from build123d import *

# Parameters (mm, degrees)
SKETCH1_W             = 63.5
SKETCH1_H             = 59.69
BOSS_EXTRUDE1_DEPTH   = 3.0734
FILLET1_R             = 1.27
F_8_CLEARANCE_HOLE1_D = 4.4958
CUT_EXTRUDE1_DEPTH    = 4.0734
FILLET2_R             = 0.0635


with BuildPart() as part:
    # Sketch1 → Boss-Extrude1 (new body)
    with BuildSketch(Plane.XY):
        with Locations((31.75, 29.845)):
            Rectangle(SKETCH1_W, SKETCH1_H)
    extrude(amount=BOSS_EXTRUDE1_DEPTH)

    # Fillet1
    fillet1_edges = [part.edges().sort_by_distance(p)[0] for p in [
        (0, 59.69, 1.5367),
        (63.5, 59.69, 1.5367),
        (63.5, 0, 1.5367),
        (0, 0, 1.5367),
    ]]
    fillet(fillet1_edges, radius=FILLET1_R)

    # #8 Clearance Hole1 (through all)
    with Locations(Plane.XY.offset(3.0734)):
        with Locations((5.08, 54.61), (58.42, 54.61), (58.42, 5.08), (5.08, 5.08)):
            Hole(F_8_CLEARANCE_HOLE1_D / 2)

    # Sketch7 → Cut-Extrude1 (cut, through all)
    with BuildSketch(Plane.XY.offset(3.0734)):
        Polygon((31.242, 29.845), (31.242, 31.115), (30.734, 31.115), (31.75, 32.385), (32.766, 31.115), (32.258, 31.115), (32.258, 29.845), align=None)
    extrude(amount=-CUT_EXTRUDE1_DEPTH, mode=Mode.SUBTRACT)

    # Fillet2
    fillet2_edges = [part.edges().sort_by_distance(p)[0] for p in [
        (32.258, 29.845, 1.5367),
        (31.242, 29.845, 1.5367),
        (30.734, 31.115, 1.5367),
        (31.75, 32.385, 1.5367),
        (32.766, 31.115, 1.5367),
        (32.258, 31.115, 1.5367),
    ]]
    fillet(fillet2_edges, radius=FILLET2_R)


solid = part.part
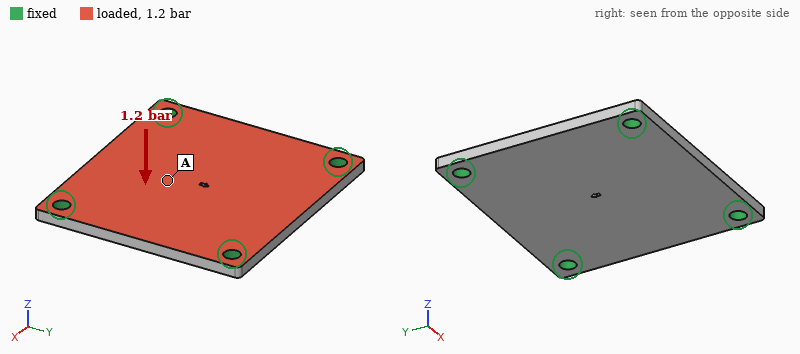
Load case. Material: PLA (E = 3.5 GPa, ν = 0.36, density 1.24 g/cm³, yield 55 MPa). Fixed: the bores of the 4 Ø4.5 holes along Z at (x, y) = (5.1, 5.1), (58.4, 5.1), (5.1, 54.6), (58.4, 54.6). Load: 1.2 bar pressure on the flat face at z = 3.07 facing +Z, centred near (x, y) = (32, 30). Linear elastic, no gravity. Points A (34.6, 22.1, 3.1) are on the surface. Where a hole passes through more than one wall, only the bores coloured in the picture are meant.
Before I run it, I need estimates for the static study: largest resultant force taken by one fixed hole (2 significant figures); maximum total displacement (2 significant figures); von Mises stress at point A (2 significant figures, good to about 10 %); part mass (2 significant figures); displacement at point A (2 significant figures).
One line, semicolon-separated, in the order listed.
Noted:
110 N; 0.61 mm; 9.9 MPa; 14 g; 0.56 mm
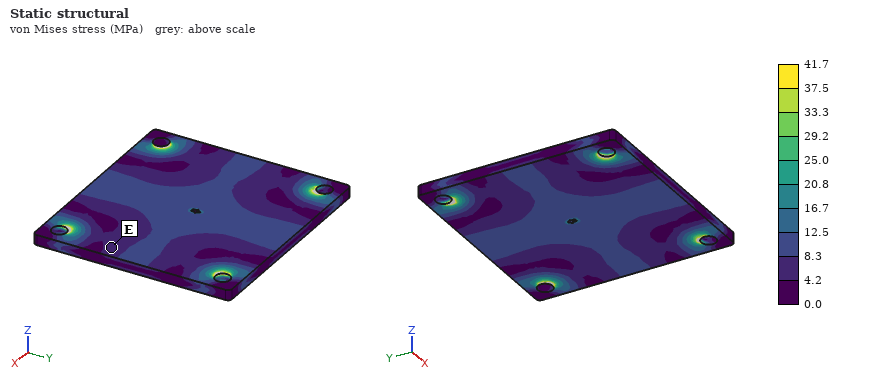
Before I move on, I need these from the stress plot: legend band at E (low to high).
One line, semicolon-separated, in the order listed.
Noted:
4.2 to 8.3 MPa
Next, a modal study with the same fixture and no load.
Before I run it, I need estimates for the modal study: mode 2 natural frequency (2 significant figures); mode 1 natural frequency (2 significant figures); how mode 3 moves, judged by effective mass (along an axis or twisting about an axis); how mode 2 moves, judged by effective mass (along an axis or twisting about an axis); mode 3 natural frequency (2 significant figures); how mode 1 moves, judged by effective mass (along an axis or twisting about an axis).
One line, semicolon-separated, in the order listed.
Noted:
2200 Hz; 1400 Hz; twisting about Y; twisting about X; 2500 Hz; along Z
